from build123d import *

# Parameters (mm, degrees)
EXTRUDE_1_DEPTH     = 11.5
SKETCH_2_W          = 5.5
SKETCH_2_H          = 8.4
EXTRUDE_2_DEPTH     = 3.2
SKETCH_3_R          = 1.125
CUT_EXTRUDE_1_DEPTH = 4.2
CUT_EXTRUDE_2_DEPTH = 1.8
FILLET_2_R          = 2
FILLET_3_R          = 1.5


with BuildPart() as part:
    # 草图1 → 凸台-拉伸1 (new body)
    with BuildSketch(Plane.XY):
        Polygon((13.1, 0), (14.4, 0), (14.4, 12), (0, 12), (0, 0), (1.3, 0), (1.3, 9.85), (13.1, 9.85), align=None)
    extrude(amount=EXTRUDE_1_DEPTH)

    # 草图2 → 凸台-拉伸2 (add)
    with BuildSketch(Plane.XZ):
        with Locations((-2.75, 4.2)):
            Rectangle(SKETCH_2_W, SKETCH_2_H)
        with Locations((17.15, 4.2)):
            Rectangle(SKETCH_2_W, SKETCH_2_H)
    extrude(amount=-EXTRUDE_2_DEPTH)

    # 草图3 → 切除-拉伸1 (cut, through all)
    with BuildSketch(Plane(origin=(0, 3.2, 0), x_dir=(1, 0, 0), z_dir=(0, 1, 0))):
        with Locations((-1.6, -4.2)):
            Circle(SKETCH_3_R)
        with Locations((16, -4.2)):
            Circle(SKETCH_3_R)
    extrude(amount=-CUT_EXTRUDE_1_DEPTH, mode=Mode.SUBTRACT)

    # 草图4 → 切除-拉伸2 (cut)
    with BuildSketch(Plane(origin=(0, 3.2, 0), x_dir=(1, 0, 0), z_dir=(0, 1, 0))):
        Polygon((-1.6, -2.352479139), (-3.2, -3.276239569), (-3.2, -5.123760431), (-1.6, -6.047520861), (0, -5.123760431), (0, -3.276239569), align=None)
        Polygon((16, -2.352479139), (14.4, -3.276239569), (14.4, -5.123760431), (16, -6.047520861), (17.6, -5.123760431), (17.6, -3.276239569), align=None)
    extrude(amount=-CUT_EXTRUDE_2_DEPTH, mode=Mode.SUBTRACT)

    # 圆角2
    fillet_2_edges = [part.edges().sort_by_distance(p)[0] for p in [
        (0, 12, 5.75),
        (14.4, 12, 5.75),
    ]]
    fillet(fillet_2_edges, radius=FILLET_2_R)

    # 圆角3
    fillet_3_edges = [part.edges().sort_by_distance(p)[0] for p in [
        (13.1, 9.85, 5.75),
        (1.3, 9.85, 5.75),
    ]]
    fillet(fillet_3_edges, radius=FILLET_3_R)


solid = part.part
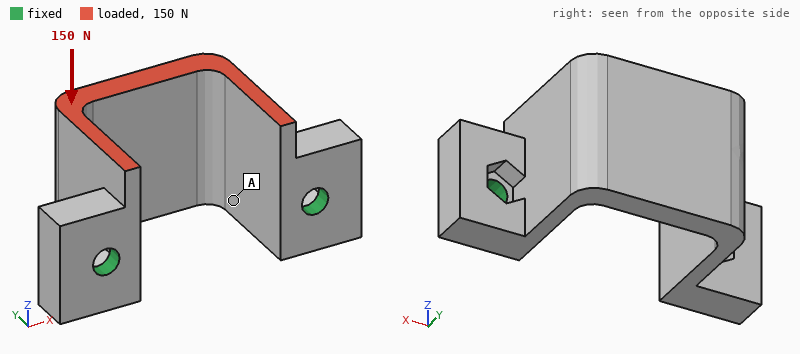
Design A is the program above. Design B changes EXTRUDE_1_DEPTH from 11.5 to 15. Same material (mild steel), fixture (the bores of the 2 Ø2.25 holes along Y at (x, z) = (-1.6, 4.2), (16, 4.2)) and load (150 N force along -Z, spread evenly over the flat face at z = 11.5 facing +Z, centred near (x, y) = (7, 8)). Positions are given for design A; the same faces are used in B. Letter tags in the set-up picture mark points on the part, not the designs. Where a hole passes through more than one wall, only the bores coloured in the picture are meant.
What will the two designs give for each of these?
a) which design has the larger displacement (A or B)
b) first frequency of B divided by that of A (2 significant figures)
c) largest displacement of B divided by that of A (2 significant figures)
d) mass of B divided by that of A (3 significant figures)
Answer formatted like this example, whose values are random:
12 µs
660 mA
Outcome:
B
0.80
1.1
1.22
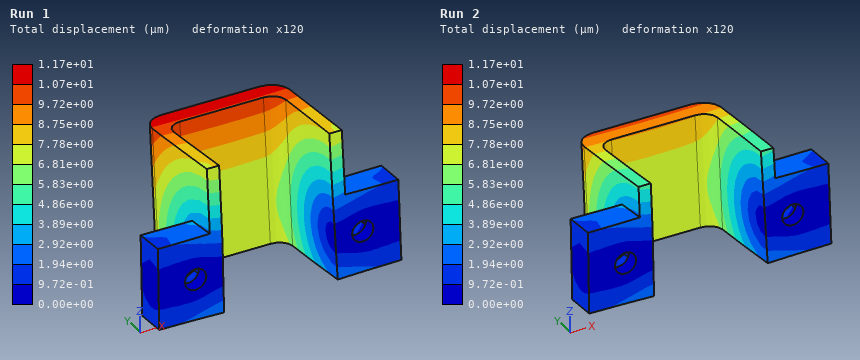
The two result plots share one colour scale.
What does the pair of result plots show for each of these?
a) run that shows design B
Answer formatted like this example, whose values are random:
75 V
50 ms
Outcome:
Run 1
